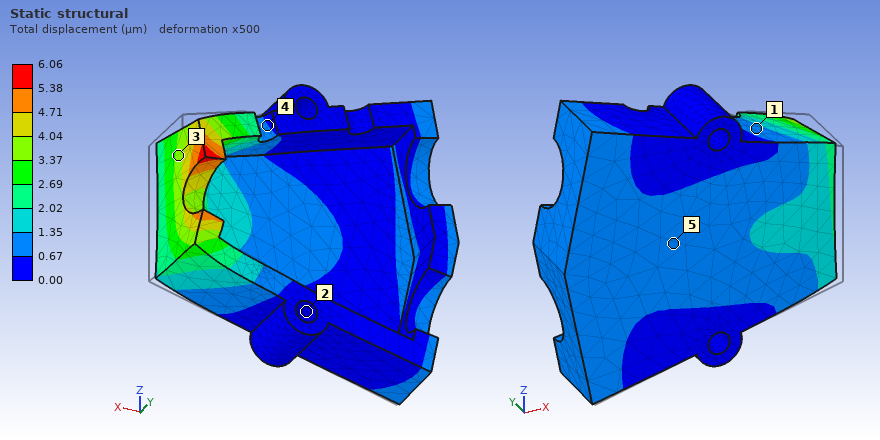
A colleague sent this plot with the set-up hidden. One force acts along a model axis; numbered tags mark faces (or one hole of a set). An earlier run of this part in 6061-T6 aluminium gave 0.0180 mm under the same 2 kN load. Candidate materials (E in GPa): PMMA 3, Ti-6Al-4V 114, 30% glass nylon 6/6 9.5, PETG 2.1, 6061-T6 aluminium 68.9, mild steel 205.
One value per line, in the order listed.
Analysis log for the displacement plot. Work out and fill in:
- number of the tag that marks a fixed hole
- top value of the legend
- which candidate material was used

2
6.06 µm
mild steel
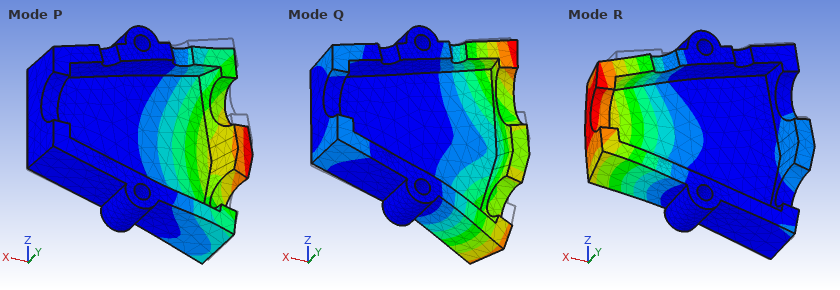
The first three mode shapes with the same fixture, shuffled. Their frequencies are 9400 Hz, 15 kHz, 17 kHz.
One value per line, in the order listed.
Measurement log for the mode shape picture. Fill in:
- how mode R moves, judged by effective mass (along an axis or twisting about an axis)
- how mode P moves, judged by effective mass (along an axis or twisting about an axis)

along Y
along Y
